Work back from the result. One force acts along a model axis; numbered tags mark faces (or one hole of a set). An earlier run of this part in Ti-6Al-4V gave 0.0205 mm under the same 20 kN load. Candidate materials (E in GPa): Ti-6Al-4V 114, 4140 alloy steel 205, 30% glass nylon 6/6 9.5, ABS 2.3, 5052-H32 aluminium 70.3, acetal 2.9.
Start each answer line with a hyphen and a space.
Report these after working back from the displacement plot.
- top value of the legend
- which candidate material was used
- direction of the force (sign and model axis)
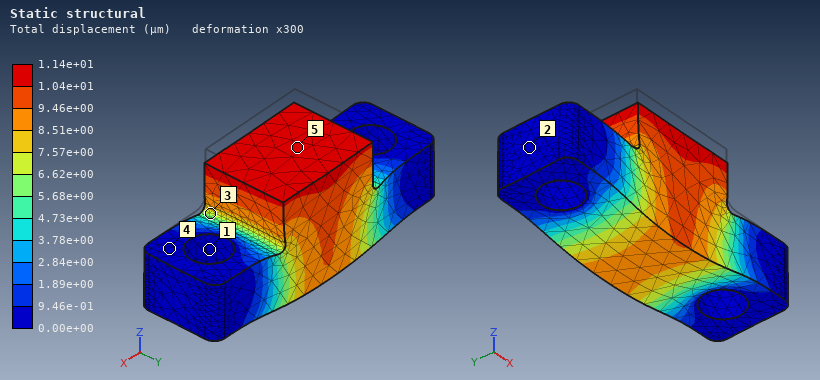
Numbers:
- 1.14e+01 µm
- 4140 alloy steel
- -Z
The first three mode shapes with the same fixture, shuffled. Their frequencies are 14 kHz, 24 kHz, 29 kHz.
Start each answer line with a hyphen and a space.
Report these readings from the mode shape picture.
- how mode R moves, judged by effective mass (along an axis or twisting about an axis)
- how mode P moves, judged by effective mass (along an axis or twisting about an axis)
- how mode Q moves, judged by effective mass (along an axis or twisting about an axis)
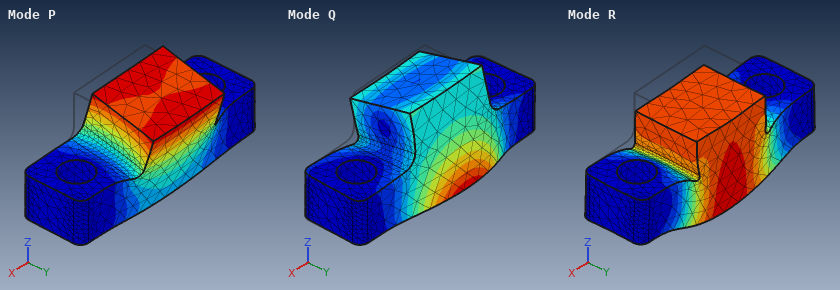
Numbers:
- along Z
- along Y
- along Y
